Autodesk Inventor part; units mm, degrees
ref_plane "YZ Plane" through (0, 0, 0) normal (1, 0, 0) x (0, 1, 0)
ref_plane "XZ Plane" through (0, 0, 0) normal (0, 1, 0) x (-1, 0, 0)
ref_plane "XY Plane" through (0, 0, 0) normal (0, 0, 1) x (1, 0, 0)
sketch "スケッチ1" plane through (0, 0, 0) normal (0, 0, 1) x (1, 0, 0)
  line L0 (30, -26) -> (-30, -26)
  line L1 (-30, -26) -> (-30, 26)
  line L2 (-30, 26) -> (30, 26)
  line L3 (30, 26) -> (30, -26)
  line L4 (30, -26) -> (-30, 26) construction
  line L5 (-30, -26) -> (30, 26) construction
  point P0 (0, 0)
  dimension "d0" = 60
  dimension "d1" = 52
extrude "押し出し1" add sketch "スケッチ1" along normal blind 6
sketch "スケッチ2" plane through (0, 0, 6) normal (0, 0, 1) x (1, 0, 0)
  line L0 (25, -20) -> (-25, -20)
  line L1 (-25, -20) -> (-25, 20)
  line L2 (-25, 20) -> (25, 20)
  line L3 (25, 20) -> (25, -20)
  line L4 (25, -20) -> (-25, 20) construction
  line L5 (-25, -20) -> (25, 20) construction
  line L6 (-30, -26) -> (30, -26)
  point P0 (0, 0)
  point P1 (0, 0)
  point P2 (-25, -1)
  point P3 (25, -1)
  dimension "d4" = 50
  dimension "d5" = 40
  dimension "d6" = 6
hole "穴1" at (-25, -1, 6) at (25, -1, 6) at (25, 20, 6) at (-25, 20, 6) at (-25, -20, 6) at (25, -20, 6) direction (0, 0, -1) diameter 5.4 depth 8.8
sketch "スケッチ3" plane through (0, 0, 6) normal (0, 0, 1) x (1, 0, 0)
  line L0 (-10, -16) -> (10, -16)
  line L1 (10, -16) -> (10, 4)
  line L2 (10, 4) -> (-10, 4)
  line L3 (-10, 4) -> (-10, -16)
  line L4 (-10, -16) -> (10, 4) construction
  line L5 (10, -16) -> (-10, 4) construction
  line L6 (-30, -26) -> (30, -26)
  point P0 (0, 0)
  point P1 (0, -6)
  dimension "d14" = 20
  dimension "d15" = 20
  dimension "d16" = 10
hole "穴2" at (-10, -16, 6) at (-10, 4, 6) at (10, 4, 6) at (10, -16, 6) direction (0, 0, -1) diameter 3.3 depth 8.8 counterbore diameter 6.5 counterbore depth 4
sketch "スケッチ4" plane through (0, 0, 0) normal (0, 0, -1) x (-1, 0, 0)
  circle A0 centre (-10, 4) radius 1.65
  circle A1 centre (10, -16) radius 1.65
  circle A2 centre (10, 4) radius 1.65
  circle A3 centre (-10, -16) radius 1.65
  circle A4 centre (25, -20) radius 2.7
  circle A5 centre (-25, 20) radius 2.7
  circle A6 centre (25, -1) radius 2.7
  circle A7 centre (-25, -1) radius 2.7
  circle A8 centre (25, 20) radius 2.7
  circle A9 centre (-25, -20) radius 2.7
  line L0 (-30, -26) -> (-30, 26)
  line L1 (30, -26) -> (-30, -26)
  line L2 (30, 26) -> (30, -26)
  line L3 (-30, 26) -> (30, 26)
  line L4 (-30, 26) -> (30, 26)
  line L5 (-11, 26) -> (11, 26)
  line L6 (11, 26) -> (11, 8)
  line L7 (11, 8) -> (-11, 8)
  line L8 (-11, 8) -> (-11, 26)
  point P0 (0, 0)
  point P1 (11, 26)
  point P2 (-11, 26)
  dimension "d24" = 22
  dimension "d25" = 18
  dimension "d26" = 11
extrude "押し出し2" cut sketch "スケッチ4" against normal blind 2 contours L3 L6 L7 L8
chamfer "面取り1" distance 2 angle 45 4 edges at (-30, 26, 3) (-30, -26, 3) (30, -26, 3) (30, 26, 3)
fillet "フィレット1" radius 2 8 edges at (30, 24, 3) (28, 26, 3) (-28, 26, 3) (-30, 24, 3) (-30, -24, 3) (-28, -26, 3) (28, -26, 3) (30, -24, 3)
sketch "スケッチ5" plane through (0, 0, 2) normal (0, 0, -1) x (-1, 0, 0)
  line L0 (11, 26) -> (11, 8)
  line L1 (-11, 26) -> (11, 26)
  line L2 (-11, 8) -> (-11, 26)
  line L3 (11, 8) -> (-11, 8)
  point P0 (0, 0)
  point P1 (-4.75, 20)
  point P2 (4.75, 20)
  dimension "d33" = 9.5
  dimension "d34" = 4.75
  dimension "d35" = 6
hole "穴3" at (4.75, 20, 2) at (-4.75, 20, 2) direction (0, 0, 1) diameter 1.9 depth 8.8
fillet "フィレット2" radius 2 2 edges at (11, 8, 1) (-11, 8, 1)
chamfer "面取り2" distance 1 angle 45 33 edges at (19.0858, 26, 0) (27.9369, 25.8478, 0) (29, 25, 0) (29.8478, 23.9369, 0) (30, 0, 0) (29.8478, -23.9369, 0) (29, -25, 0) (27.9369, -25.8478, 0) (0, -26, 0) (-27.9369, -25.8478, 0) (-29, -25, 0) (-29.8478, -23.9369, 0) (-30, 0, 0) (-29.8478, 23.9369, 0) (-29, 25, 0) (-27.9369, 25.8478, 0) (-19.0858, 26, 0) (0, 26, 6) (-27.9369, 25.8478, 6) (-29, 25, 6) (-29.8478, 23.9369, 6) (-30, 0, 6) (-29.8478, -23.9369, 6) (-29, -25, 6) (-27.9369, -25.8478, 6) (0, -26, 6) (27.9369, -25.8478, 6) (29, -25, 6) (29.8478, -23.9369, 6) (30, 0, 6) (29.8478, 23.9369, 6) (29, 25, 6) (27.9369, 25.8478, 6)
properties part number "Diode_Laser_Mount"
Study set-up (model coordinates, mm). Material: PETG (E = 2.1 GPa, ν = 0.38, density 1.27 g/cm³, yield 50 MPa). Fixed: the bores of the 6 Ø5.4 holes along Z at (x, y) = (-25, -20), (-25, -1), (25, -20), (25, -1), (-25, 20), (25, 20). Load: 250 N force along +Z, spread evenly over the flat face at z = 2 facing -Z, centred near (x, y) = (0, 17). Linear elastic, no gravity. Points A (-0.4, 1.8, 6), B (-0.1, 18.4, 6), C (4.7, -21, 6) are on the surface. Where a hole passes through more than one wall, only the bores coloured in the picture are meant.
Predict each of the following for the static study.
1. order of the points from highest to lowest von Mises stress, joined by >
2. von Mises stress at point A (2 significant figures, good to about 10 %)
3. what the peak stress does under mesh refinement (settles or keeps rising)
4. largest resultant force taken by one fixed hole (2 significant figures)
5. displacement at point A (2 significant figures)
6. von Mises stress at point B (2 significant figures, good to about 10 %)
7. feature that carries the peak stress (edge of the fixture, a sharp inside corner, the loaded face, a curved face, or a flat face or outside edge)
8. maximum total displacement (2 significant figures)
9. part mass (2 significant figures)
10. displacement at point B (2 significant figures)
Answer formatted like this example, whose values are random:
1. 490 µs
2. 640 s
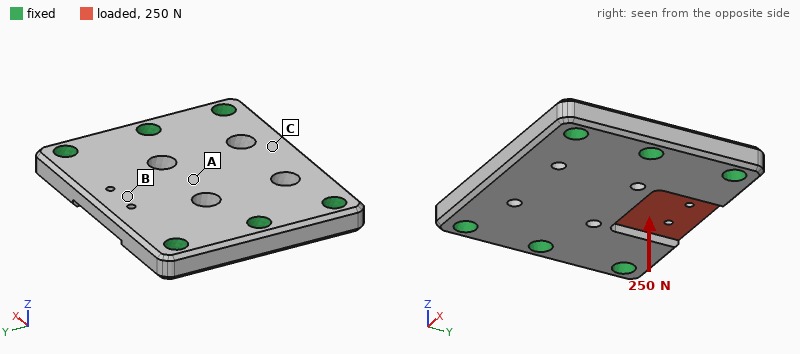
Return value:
1. B > A > C
2. 2.8 MPa
3. keeps rising
4. 120 N
5. 0.083 mm
6. 8.3 MPa
7. edge of the fixture
8. 0.29 mm
9. 21 g
10. 0.22 mm
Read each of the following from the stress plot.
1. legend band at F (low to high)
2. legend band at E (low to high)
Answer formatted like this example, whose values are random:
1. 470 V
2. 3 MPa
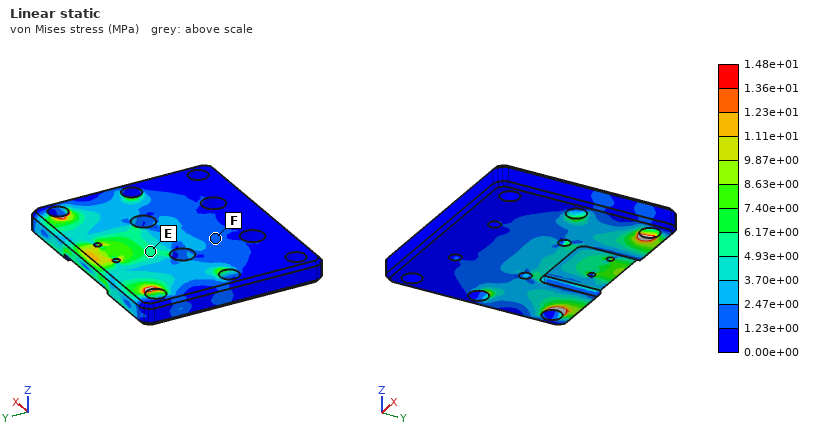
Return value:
1. 1.23e+00 to 2.47e+00 MPa
2. 4.93e+00 to 6.17e+00 MPa
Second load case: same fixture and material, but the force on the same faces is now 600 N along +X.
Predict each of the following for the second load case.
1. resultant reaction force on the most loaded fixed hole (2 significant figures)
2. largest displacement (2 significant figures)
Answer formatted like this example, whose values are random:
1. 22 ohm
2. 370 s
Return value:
1. 200 N
2. 45 µm
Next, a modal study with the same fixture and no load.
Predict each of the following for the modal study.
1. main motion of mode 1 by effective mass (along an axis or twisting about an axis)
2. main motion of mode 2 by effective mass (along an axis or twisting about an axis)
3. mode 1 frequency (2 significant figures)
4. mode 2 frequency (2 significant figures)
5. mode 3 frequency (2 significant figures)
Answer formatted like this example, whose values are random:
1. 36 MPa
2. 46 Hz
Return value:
1. along Z
2. twisting about X
3. 3200 Hz
4. 3700 Hz
5. 5400 Hz
